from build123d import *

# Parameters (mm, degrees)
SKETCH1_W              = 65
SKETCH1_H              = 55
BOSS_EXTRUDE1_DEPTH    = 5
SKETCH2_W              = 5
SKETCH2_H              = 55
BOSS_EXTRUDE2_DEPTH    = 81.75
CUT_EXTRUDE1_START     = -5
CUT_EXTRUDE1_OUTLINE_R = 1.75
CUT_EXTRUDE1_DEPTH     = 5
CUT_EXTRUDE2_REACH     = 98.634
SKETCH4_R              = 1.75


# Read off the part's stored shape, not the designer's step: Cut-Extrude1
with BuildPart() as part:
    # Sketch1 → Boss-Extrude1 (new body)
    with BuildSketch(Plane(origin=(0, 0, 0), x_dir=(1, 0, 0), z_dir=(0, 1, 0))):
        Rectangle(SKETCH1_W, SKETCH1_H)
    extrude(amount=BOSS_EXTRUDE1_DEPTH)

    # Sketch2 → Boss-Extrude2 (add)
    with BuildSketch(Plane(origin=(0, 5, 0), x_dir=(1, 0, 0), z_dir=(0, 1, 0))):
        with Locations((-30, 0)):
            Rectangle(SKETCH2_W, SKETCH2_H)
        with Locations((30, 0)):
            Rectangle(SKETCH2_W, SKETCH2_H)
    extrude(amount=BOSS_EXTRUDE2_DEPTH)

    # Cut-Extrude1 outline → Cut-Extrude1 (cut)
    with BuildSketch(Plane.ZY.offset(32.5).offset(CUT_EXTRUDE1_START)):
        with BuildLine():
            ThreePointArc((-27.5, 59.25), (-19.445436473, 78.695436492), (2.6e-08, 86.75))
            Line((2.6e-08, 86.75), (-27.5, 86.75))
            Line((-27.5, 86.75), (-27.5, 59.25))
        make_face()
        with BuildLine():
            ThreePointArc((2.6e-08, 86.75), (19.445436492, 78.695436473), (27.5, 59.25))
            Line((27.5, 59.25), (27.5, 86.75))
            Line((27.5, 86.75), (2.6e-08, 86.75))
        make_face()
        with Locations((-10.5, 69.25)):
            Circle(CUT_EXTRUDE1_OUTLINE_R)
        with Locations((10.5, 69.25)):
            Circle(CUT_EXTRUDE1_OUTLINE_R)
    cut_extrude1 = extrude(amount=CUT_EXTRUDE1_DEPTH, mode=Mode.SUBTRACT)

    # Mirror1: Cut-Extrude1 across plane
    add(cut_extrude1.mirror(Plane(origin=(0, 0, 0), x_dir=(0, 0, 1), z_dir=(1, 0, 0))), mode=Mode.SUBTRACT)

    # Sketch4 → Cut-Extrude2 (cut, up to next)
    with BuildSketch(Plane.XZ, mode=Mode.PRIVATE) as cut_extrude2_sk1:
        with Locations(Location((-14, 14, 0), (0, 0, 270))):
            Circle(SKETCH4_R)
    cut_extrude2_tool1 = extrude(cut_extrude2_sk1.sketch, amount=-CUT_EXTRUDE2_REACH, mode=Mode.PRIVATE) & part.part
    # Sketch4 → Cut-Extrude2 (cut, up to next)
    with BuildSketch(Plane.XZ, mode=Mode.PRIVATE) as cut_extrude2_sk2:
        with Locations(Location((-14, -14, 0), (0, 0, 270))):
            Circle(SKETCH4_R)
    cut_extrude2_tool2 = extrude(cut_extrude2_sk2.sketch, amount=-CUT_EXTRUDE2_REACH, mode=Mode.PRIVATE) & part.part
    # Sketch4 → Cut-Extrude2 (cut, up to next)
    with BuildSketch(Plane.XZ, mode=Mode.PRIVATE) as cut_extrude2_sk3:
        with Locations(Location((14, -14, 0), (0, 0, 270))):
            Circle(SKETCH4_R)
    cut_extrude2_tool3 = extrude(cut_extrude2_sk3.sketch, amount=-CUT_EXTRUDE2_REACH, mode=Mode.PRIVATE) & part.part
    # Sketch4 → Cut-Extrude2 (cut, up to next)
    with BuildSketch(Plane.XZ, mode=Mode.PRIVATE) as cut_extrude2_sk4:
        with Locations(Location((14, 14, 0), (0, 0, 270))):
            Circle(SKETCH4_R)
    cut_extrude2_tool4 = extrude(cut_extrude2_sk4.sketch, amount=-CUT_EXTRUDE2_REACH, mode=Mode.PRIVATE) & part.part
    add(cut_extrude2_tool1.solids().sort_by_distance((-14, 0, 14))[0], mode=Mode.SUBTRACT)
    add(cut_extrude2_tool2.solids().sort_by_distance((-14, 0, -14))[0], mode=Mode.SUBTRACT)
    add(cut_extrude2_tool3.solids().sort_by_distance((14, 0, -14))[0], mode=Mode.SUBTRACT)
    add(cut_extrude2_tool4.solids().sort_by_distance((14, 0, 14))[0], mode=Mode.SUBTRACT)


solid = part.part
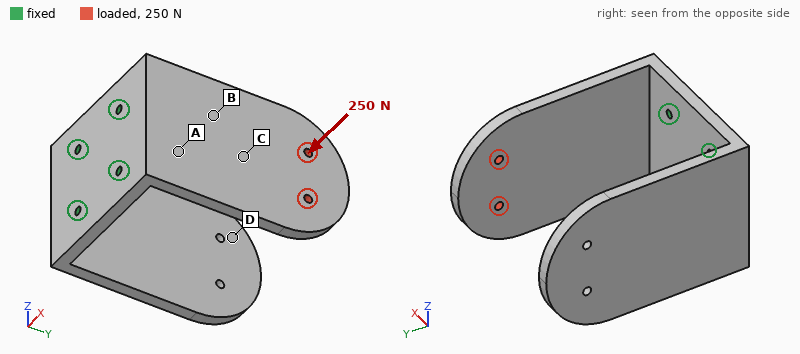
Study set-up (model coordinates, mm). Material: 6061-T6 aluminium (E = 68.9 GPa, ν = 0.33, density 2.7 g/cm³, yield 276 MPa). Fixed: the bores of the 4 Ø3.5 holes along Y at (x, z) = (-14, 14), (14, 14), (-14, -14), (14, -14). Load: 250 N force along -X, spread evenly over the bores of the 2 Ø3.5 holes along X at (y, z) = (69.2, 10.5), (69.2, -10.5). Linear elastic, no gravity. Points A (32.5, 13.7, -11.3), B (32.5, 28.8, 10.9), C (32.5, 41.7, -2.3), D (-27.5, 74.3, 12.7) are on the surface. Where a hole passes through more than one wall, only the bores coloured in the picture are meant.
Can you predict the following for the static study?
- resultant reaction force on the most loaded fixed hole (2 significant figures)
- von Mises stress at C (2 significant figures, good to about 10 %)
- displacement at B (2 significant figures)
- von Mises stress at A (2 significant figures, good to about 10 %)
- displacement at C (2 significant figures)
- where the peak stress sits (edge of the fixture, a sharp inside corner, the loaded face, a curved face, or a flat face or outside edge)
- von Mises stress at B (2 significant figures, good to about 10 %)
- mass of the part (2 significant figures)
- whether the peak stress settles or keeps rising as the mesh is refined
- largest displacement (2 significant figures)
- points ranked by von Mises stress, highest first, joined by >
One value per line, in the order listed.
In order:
170 N
28 MPa
0.30 mm
54 MPa
0.50 mm
edge of the fixture
40 MPa
160 g
keeps rising
1.4 mm
A > B > C > D
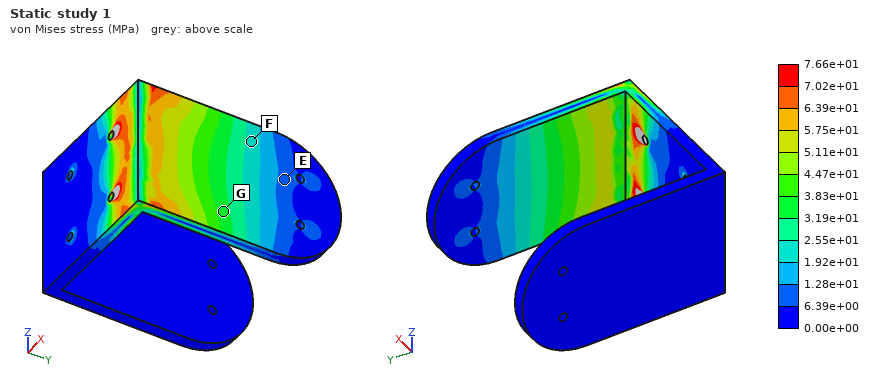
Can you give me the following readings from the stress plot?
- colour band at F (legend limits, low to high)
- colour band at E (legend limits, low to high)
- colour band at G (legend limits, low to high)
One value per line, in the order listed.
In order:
1.92e+01 to 2.55e+01 MPa
6.39e+00 to 1.28e+01 MPa
3.19e+01 to 3.83e+01 MPa
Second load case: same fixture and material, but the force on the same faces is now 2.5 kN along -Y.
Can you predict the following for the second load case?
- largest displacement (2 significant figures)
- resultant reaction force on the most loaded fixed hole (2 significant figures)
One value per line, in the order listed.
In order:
0.79 mm
1.5 kN
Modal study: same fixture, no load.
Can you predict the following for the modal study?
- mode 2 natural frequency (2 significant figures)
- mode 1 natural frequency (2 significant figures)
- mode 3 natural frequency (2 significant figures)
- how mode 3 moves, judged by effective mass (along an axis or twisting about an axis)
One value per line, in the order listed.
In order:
510 Hz
500 Hz
1400 Hz
along Z
